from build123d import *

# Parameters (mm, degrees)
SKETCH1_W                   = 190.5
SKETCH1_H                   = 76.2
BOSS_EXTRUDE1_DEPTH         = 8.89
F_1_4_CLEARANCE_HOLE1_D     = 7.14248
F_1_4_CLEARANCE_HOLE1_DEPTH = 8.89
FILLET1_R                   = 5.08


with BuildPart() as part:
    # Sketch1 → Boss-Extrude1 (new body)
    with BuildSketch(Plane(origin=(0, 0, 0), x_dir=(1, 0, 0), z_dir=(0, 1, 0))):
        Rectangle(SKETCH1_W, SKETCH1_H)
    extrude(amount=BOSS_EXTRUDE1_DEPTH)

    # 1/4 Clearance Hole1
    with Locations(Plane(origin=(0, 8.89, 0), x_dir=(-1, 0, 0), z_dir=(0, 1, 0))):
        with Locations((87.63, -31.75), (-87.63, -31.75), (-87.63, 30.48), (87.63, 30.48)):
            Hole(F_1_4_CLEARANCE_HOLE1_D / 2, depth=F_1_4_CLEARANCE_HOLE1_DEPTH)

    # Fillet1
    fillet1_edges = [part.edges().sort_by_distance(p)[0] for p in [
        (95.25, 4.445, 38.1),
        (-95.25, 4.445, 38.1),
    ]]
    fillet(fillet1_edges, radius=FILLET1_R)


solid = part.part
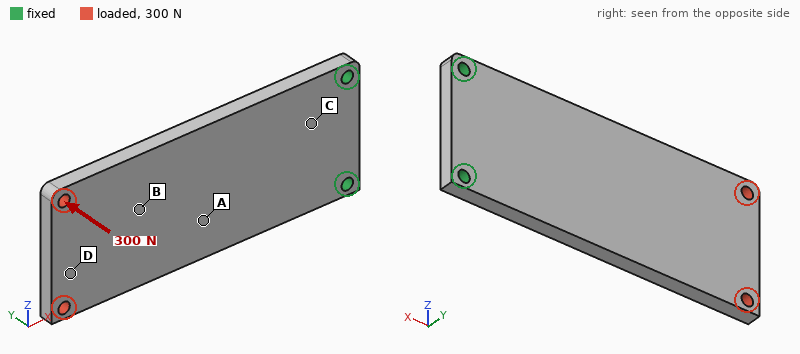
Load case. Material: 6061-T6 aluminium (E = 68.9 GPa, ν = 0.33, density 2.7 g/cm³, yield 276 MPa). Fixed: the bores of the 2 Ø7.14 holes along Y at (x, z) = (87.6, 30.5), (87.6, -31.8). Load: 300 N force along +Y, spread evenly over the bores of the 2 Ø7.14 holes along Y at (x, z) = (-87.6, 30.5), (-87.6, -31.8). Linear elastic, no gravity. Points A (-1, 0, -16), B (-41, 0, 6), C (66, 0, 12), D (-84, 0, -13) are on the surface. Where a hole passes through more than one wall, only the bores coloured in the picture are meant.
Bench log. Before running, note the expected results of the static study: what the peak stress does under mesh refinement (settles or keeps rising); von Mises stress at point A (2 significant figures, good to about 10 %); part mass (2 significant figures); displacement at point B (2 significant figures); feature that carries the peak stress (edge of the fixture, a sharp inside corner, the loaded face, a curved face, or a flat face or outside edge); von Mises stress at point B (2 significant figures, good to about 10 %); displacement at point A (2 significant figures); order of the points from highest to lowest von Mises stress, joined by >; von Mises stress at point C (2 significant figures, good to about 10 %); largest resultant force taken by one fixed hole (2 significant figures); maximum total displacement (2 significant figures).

keeps rising
26 MPa
340 g
1.2 mm
edge of the fixture
14 MPa
0.65 mm
C > A > B > D
41 MPa
160 N
2.0 mm
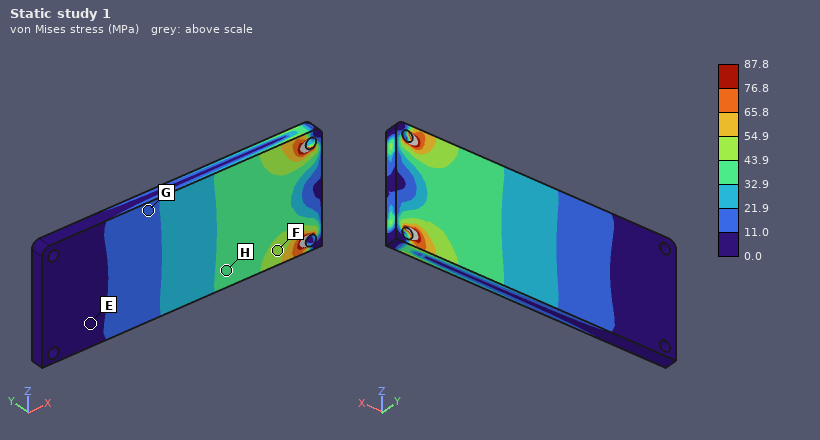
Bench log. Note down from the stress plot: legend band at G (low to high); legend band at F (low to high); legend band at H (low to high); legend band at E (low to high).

11.0 to 21.9 MPa
43.9 to 54.9 MPa
32.9 to 43.9 MPa
0.0 to 11.0 MPa
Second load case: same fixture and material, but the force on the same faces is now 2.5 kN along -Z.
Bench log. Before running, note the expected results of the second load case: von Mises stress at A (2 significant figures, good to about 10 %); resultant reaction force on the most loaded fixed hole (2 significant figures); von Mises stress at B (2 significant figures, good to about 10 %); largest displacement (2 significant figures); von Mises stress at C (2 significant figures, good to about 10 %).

13 MPa
7.1 kN
9.7 MPa
0.25 mm
13 MPa
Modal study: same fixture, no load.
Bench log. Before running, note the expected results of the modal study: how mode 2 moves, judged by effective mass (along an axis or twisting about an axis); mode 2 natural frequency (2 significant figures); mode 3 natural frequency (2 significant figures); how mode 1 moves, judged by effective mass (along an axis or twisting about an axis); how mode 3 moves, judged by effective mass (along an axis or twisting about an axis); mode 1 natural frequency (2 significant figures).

twisting about X
1100 Hz
1300 Hz
along Y
along Y
210 Hz
